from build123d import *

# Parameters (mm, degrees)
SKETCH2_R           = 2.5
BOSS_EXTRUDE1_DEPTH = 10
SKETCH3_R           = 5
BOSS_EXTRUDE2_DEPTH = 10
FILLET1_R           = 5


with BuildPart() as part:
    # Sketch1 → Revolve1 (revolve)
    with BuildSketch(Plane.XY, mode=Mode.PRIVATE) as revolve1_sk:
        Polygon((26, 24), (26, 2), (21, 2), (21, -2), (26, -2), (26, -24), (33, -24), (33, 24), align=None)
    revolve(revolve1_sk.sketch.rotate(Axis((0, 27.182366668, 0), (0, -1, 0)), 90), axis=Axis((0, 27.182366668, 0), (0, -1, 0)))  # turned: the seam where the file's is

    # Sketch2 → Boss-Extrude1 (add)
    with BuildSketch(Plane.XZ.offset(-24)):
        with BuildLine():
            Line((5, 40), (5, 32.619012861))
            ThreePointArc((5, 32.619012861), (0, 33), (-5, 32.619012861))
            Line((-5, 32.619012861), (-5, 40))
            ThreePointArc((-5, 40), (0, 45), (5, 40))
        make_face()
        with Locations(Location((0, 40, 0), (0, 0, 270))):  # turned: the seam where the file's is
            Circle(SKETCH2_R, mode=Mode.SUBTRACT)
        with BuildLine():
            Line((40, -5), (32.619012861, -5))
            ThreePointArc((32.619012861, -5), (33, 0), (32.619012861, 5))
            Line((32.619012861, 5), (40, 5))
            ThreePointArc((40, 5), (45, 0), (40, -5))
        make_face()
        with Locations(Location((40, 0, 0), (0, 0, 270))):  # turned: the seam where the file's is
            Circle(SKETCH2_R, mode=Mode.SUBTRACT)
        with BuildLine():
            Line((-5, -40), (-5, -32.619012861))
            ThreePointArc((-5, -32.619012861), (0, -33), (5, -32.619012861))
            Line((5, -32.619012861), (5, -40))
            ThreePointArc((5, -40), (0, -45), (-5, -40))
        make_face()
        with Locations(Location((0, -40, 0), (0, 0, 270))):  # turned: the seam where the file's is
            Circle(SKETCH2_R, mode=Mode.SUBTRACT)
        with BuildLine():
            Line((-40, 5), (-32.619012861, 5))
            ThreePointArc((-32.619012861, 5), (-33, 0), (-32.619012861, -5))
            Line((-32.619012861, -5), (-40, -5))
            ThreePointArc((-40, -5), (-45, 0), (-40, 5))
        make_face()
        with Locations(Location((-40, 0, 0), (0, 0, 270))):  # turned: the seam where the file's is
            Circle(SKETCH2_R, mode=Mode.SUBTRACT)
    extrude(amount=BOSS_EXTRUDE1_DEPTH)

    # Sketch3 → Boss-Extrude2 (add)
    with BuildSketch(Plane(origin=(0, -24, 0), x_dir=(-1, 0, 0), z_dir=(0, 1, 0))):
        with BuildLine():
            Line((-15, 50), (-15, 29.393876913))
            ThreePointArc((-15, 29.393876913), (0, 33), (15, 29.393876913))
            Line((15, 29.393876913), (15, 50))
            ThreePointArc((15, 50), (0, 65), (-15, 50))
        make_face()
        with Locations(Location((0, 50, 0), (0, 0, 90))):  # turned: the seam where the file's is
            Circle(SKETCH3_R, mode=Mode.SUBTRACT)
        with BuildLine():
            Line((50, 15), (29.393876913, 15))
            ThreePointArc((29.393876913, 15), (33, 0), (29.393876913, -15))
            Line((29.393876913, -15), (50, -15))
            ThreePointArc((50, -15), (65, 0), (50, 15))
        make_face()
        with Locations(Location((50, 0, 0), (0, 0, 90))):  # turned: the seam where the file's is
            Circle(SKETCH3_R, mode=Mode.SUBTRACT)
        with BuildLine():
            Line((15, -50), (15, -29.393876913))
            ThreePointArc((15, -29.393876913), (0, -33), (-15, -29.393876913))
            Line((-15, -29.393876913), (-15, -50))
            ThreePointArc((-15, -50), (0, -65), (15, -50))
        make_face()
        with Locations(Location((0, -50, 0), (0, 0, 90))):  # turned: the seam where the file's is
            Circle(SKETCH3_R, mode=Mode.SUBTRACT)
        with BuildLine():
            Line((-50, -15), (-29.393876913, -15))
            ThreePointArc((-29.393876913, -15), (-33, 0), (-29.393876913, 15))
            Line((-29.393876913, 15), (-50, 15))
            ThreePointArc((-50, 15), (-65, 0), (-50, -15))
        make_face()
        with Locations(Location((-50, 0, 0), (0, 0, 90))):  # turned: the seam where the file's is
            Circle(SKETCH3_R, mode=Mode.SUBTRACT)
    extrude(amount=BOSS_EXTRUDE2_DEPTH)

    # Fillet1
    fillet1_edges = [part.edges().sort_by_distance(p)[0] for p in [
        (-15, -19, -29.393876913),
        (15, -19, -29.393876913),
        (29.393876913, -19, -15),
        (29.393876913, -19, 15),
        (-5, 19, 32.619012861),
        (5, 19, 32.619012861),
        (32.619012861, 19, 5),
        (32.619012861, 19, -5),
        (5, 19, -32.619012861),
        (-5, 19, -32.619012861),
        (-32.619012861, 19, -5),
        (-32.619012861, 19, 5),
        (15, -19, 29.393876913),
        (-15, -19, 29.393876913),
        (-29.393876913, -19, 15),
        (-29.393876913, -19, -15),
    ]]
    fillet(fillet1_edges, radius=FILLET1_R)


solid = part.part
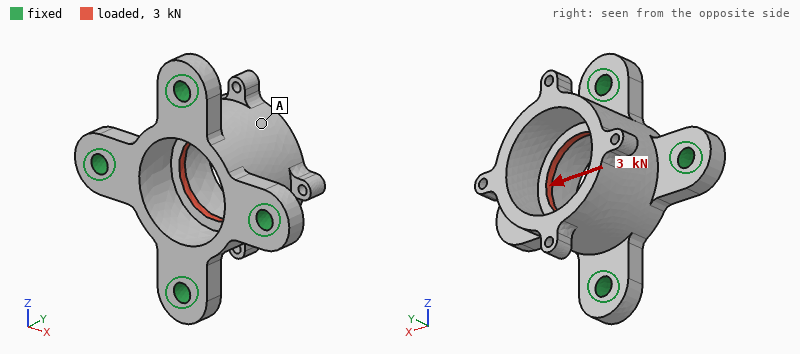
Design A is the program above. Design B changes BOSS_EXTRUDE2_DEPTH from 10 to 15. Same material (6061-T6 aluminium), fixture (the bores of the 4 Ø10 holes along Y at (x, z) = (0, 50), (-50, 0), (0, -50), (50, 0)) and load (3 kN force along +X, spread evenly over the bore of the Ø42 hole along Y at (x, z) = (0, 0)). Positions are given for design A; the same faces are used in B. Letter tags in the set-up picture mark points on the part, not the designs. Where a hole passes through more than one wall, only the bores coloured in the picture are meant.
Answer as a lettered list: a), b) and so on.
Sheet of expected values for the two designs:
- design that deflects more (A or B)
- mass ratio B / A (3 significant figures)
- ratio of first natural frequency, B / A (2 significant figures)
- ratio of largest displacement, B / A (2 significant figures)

a) A
b) 1.16
c) 1.3
d) 0.53
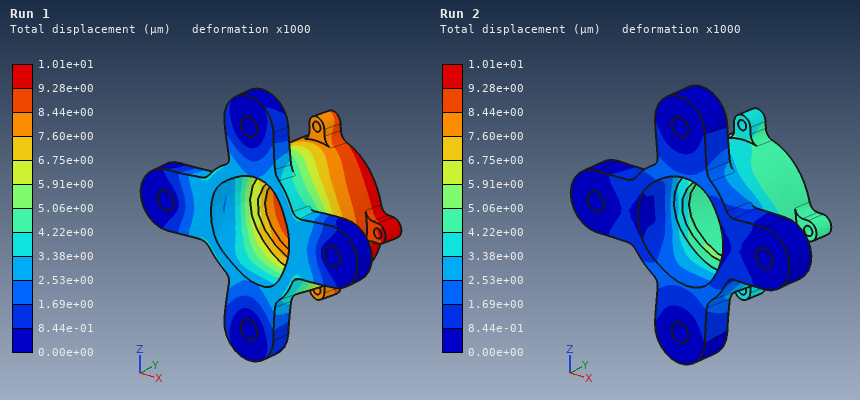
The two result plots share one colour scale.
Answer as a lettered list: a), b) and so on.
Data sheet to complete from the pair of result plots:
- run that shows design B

a) Run 2
